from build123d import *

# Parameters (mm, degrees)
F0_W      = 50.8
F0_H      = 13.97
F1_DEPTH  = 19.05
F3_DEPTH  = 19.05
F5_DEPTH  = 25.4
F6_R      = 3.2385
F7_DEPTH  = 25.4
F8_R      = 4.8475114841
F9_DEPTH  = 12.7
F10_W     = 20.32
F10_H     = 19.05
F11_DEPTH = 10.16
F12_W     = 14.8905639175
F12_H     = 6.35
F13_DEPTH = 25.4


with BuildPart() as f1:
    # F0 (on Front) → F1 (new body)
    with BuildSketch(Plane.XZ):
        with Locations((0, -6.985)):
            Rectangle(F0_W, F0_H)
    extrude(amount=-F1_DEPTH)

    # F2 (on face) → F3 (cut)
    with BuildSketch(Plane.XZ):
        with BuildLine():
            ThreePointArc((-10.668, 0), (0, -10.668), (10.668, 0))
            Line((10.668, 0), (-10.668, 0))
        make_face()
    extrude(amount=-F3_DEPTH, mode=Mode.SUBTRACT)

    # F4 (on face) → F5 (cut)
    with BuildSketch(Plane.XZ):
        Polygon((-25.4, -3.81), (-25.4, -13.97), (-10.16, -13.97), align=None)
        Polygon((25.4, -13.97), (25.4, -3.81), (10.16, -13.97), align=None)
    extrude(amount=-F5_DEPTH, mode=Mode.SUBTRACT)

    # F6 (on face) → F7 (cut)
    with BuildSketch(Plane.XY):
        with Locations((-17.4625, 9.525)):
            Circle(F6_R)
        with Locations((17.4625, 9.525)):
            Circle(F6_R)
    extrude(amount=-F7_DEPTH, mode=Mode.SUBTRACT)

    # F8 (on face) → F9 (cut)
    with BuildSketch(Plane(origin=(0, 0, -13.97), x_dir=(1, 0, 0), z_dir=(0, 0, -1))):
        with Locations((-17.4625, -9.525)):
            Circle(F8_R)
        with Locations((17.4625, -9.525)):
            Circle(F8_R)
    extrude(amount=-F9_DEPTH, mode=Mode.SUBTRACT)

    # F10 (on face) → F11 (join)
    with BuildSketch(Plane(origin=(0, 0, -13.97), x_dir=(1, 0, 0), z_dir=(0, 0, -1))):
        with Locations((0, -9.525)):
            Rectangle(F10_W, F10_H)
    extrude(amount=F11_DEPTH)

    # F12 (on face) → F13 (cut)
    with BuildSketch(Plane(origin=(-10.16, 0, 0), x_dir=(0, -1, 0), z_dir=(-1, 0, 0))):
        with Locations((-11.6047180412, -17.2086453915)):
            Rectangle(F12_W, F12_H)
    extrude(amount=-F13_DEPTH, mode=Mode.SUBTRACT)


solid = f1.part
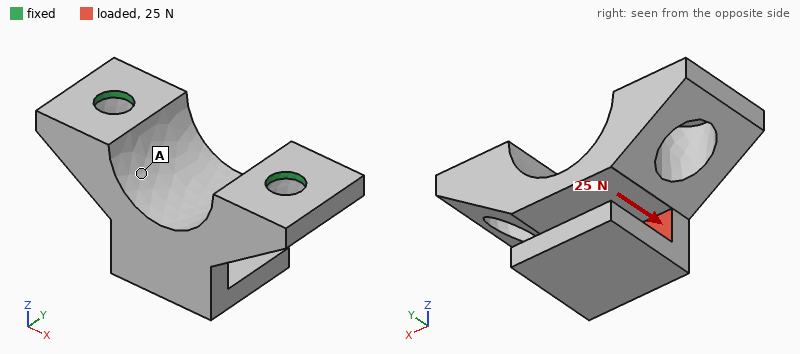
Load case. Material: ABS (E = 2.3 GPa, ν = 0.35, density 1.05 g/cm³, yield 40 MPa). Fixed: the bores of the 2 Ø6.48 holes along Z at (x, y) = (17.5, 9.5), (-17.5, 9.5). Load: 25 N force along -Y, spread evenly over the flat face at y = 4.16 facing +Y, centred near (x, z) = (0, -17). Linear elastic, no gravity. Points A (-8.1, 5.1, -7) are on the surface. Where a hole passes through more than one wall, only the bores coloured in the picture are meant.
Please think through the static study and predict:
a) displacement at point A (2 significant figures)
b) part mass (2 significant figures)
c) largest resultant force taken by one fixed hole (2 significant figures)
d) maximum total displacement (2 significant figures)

0.037 mm
8.3 g
13 N
0.14 mm
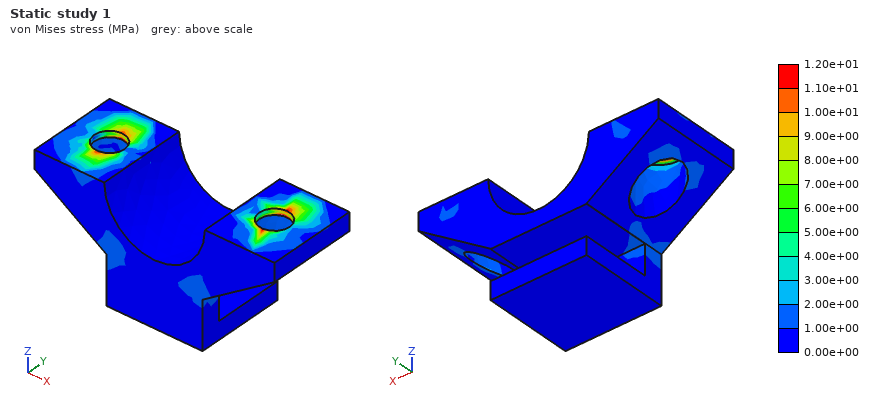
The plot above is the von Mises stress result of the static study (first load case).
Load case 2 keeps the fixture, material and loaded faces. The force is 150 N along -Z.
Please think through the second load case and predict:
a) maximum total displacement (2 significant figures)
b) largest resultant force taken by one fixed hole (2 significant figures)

0.18 mm
92 N
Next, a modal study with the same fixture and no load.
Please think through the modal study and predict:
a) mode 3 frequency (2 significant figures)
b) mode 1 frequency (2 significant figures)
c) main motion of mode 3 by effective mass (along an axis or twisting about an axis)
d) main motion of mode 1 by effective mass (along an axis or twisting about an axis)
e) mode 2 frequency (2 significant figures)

2500 Hz
1100 Hz
along X
along Y
2000 Hz
